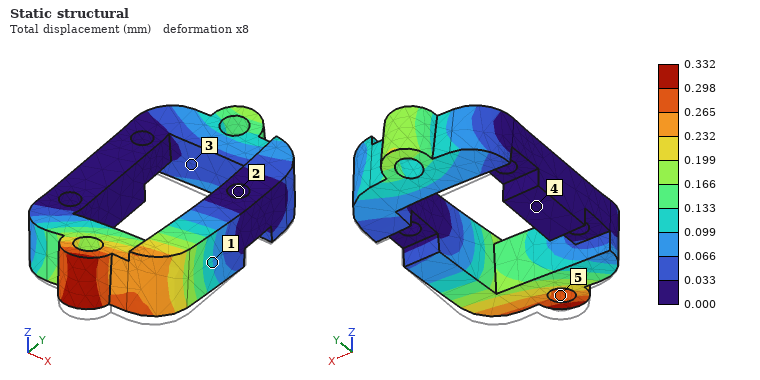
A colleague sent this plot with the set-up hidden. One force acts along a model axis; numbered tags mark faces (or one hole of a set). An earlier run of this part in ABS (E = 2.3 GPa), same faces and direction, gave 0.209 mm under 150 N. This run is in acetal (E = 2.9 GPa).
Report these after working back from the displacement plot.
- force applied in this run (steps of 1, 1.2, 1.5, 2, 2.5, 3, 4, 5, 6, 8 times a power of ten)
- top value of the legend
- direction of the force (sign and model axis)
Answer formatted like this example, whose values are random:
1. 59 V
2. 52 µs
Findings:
1. 300 N
2. 0.332 mm
3. +Z
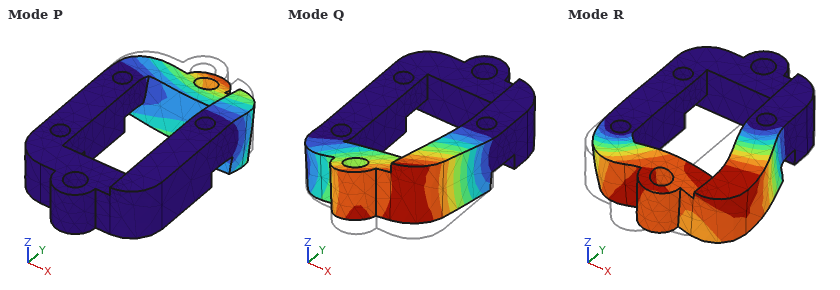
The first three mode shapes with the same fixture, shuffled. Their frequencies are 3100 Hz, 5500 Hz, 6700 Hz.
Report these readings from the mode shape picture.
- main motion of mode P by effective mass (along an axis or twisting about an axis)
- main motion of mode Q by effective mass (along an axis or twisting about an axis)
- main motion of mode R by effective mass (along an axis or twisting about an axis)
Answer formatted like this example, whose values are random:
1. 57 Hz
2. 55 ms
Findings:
1. along Z
2. along Z
3. along X
